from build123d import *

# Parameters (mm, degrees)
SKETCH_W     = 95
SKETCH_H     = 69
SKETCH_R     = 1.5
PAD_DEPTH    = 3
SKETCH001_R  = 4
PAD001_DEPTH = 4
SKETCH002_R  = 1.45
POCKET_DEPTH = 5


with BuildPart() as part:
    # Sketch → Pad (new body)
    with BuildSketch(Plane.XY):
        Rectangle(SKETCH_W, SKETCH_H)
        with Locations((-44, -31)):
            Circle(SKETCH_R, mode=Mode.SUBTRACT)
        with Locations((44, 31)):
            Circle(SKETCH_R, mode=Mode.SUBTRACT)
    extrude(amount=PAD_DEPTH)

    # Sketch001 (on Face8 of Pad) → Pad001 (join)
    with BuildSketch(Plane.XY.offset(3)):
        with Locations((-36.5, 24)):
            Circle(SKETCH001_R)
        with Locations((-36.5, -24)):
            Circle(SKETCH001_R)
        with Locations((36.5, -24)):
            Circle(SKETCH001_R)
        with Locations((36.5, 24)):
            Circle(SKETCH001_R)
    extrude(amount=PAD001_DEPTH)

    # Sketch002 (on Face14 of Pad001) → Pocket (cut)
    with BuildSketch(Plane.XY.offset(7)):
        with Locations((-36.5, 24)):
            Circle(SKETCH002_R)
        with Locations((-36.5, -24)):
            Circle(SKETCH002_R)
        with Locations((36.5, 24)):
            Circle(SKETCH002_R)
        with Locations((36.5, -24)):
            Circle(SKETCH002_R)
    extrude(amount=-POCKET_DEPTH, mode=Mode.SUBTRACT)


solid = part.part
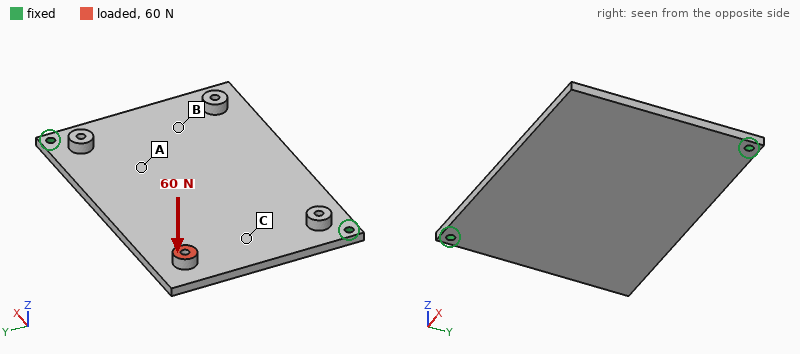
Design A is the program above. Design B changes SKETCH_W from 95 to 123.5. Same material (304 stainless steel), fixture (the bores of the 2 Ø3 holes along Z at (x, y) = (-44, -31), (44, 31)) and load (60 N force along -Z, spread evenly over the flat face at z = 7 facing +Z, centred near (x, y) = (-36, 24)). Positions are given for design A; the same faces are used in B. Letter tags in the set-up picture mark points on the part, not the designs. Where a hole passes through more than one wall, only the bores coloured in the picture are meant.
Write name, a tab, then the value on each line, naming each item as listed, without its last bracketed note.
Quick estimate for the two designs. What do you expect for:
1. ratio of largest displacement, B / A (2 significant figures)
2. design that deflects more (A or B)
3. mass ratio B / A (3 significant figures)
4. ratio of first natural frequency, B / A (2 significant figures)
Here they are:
ratio of largest displacement, B / A	0.81
design that deflects more	A
mass ratio B / A	1.29
ratio of first natural frequency, B / A	0.93
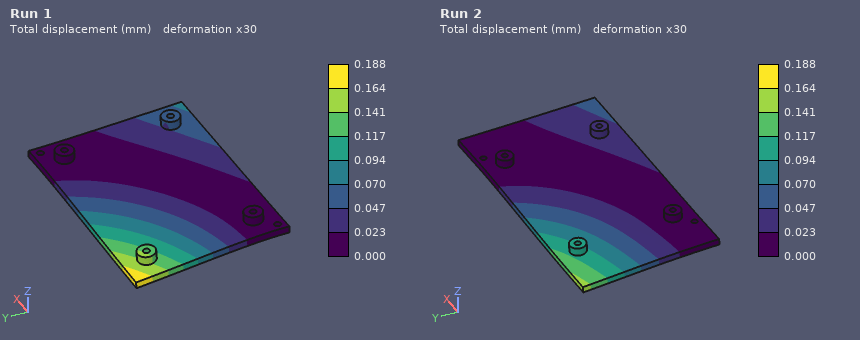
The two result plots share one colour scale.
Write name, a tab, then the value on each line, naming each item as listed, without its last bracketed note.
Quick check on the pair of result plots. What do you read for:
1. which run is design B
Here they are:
which run is design B	Run 2
